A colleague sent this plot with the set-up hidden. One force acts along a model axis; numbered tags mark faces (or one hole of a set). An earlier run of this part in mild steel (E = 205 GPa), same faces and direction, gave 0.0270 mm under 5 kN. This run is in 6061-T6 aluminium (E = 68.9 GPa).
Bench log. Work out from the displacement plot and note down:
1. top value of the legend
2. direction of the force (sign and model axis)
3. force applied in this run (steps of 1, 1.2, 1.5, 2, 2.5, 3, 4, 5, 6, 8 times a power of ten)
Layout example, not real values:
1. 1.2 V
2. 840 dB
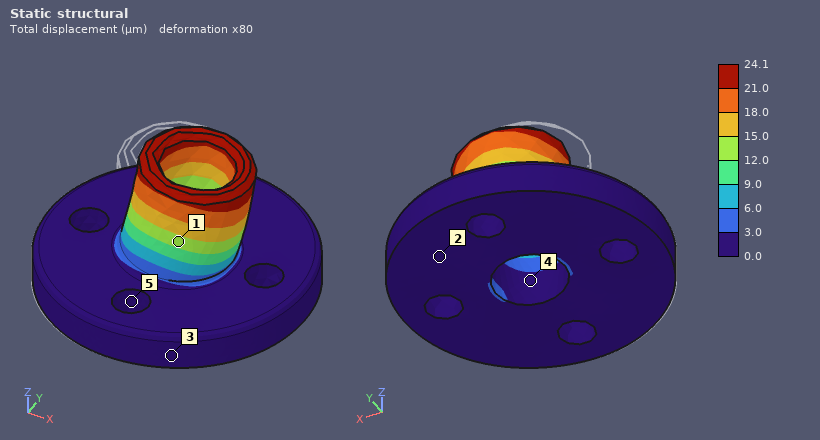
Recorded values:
1. 24.1 µm
2. +X
3. 1.5 kN
